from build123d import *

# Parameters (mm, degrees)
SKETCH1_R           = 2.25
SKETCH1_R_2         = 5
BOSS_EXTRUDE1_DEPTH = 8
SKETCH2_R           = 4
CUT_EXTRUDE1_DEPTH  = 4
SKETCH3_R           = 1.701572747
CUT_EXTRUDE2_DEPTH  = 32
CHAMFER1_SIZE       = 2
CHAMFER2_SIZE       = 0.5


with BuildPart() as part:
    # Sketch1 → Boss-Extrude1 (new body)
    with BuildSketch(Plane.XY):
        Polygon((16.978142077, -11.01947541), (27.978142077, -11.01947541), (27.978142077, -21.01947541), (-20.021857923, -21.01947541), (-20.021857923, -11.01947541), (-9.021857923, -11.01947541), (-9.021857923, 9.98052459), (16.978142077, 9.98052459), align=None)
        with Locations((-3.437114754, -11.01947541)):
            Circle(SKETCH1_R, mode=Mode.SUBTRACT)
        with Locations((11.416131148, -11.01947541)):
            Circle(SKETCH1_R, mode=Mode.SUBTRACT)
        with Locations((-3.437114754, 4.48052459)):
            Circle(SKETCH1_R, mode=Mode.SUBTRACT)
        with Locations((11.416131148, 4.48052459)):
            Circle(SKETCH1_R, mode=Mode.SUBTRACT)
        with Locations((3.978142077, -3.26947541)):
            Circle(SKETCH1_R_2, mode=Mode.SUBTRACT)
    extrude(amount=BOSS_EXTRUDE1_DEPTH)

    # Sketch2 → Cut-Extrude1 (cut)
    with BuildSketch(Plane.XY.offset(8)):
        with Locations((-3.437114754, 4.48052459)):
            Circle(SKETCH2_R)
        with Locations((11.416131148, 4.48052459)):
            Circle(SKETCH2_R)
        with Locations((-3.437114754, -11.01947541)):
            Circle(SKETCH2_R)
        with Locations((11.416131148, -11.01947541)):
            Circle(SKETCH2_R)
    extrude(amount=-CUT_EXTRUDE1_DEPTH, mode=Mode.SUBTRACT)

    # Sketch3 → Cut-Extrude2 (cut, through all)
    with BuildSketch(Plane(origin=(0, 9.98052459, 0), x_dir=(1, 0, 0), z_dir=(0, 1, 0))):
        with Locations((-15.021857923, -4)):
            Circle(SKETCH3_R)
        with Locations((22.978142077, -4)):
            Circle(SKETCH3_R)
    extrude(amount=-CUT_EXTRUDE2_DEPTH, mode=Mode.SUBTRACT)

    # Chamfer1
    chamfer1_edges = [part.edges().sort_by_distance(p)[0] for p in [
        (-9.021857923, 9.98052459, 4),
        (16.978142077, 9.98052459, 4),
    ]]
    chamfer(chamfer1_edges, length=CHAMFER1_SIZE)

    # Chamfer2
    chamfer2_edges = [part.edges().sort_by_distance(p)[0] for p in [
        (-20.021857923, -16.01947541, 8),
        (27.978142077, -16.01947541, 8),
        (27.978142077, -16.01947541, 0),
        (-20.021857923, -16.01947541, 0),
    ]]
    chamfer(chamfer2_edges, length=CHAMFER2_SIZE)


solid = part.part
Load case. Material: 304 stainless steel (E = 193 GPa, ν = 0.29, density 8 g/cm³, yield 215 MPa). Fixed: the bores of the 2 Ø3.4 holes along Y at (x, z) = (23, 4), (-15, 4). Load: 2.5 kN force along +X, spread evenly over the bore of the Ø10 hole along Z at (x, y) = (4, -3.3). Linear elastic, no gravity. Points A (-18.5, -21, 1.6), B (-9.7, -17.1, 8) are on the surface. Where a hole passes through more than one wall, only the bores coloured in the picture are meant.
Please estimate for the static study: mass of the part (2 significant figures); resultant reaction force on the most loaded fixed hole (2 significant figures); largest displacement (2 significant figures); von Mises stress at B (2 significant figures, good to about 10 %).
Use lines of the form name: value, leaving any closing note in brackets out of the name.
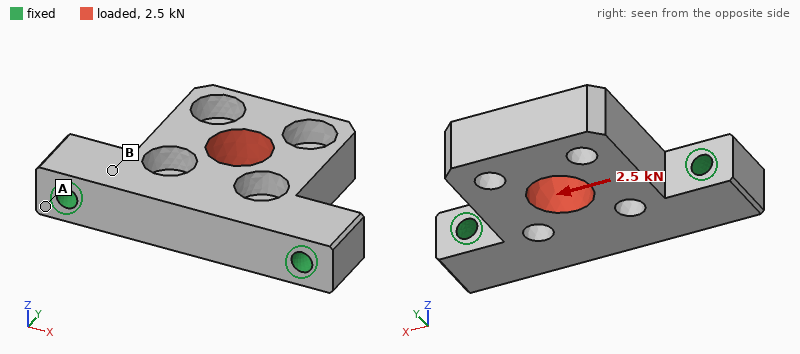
mass of the part: 50 g
resultant reaction force on the most loaded fixed hole: 1.6 kN
largest displacement: 9.8 µm
von Mises stress at B: 15 MPa
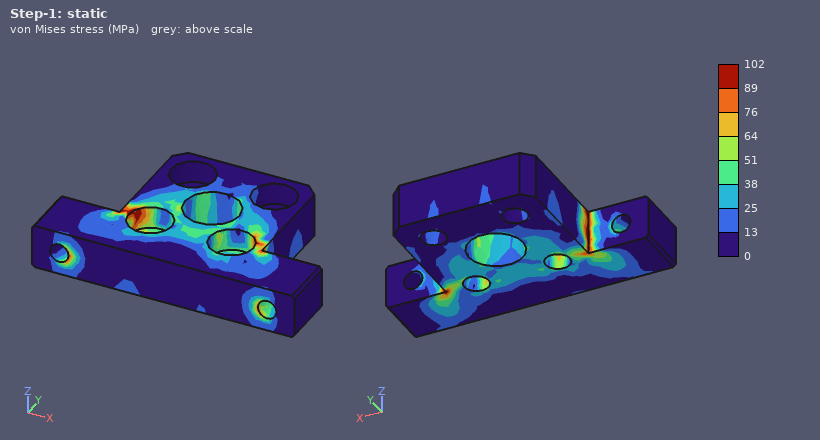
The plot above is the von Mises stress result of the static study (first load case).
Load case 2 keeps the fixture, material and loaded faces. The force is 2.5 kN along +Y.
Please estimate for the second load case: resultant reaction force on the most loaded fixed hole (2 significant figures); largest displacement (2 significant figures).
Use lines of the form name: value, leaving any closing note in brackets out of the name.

resultant reaction force on the most loaded fixed hole: 1.3 kN
largest displacement: 6.4 µm
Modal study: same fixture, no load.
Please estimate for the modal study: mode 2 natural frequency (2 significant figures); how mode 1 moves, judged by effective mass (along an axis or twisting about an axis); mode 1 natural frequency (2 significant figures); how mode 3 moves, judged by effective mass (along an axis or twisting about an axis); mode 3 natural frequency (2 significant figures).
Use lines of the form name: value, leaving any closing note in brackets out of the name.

mode 2 natural frequency: 14 kHz
how mode 1 moves, judged by effective mass: along Z
mode 1 natural frequency: 5400 Hz
how mode 3 moves, judged by effective mass: along X
mode 3 natural frequency: 16 kHz
